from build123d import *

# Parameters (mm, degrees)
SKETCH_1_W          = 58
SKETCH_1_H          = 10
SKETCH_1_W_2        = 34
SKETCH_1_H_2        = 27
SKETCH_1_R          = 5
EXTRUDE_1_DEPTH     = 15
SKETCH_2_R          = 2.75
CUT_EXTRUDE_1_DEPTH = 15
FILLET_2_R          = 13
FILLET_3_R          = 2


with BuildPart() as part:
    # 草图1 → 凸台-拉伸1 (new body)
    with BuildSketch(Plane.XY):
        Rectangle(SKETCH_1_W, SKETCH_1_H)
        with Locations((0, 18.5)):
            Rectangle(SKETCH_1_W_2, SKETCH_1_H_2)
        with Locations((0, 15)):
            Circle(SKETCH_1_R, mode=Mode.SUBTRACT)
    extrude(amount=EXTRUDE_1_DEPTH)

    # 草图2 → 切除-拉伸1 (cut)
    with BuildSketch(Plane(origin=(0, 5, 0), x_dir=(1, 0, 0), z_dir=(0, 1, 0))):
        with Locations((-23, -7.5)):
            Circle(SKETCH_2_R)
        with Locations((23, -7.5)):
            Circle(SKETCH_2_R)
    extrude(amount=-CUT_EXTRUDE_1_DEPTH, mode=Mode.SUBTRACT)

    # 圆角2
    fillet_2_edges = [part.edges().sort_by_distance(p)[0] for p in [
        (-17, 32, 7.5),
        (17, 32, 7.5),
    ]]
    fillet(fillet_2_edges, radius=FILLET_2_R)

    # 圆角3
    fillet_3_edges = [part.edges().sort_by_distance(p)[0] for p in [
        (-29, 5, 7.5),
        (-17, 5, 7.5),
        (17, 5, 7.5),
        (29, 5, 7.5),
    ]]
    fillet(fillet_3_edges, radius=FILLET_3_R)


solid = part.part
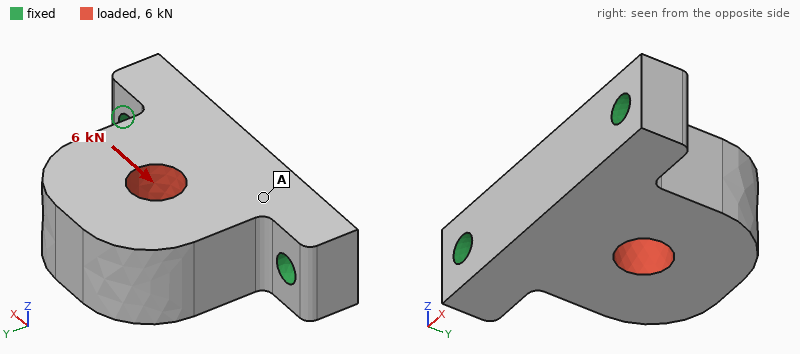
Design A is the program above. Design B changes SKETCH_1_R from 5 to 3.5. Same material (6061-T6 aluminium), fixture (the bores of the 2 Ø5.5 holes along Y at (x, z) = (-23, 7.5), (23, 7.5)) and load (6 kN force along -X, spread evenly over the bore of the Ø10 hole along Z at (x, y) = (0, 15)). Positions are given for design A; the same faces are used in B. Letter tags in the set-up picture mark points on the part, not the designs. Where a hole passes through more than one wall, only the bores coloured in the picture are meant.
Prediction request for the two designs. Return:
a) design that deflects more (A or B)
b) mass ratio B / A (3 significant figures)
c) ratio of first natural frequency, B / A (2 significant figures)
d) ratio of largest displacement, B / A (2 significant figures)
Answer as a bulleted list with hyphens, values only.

- A
- 1.03
- 0.99
- 0.92
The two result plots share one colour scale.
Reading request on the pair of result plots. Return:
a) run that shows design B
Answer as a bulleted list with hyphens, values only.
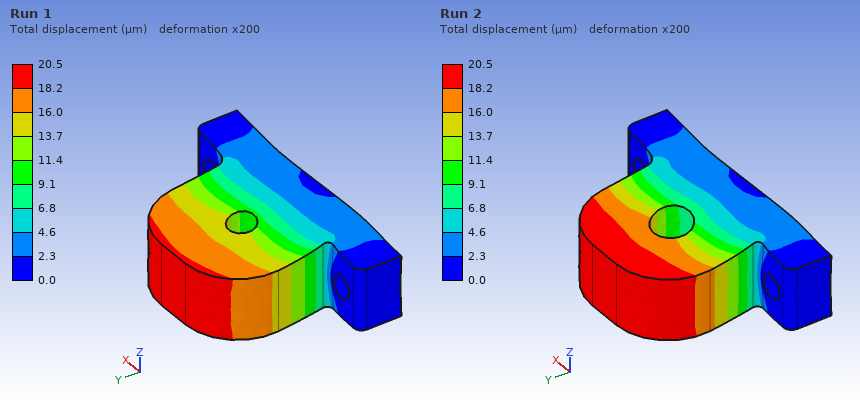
- Run 1
